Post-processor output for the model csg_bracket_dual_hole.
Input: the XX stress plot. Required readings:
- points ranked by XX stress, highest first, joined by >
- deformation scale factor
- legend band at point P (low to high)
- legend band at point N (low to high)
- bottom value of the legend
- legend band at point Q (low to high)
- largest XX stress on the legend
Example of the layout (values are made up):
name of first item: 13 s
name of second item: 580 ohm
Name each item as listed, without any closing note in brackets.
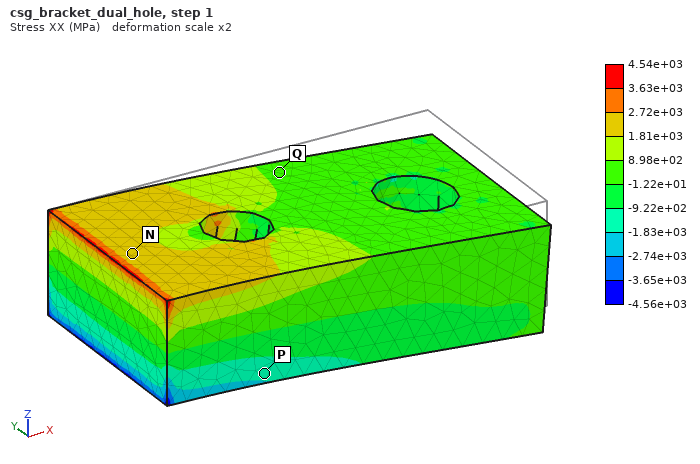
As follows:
points ranked by XX stress, highest first, joined by >: N > Q > P
deformation scale factor: 2
legend band at point P: -1.83e+03 to -9.22e+02 MPa
legend band at point N: 1.81e+03 to 2.72e+03 MPa
bottom value of the legend: -4.56e+03 MPa
legend band at point Q: -1.22e+01 to 8.98e+02 MPa
largest XX stress on the legend: 4.54e+03 MPa
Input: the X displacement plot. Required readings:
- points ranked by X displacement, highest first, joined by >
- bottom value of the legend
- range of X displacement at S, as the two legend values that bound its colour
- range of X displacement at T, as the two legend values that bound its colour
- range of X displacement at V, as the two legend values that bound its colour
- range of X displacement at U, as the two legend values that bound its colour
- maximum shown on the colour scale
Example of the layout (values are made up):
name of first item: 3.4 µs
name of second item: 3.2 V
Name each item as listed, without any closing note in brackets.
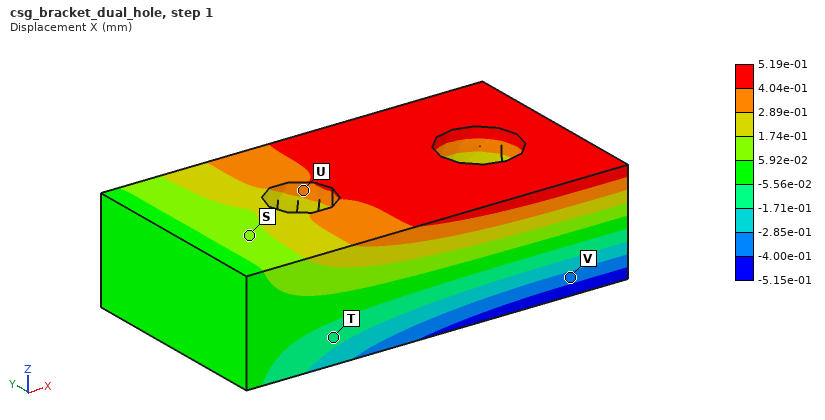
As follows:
points ranked by X displacement, highest first, joined by >: U > S > T > V
bottom value of the legend: -5.15e-01 mm
range of X displacement at S, as the two legend values that bound its colour: 5.92e-02 to 1.74e-01 mm
range of X displacement at T, as the two legend values that bound its colour: -1.71e-01 to -5.56e-02 mm
range of X displacement at V, as the two legend values that bound its colour: -4.00e-01 to -2.85e-01 mm
range of X displacement at U, as the two legend values that bound its colour: 2.89e-01 to 4.04e-01 mm
maximum shown on the colour scale: 5.19e-01 mm
